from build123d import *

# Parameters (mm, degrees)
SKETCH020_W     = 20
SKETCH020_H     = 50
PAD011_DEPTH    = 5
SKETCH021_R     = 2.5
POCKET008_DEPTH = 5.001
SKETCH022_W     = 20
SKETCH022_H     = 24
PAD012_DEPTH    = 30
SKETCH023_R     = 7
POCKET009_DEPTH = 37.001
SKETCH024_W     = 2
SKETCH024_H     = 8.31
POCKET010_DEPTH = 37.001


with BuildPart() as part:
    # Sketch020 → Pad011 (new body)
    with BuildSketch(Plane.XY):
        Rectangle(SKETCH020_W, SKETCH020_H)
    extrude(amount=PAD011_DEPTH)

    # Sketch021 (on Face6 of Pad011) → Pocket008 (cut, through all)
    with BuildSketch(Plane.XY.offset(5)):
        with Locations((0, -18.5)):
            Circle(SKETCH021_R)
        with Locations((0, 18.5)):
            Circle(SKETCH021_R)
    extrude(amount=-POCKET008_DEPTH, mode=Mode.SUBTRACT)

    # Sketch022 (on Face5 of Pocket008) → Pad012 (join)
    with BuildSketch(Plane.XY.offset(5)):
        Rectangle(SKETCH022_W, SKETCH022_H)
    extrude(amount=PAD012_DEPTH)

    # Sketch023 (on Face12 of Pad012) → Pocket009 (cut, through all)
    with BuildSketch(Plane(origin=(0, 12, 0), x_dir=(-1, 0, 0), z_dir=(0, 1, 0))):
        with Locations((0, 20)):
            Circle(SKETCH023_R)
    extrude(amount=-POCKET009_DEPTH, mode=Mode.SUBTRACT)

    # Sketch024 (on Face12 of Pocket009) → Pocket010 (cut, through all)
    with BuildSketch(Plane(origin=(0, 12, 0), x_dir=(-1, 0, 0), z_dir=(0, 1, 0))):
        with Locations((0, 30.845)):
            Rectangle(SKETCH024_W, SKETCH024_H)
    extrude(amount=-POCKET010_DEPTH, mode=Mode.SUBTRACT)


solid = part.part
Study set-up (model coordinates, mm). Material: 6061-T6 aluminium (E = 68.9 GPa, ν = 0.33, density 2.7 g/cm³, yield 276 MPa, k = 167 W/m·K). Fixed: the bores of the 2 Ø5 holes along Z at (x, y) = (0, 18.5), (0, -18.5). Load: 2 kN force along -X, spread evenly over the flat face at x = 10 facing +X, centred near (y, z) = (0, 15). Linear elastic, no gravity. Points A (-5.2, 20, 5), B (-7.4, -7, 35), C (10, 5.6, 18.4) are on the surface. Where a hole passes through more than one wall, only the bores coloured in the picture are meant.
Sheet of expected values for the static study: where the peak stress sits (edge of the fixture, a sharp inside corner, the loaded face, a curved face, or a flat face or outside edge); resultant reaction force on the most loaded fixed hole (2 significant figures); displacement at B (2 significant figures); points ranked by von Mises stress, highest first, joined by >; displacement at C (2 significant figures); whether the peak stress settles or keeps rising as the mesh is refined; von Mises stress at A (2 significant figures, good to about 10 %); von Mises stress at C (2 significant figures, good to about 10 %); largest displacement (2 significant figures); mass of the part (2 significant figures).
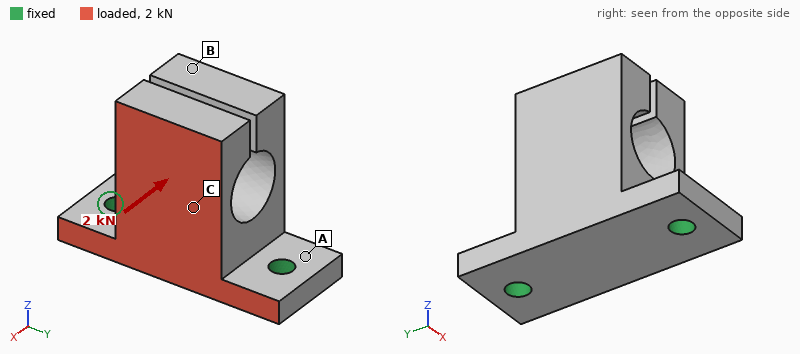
edge of the fixture
1.0 kN
0.14 mm
C > A > B
0.11 mm
keeps rising
51 MPa
140 MPa
0.36 mm
41 g
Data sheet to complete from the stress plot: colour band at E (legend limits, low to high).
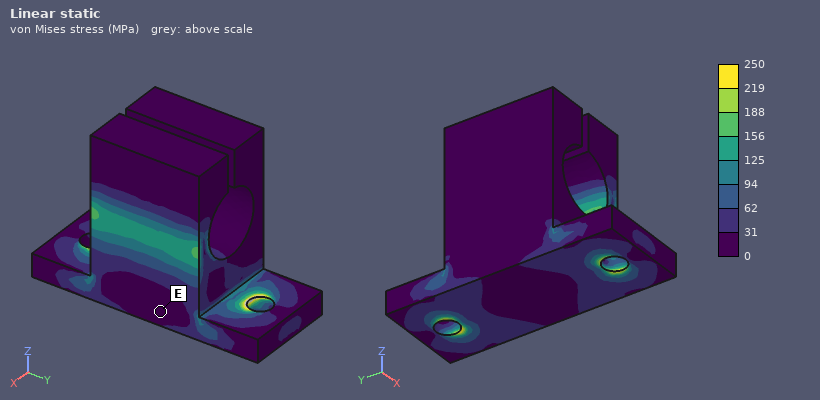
0 to 31 MPa
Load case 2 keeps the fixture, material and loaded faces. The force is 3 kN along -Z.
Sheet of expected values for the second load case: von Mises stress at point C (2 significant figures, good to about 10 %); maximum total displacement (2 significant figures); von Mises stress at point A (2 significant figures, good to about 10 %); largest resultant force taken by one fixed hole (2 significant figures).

57 MPa
0.23 mm
42 MPa
1.6 kN
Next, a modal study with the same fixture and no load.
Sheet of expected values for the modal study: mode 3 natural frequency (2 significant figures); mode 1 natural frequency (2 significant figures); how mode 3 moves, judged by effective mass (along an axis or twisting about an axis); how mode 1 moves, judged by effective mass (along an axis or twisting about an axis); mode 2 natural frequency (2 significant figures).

7800 Hz
2800 Hz
along Y
along X
3900 Hz
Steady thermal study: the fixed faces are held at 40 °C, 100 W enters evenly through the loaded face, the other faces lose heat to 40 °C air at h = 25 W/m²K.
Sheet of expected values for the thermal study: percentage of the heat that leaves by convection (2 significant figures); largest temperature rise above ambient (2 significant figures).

4.0 %
79 K
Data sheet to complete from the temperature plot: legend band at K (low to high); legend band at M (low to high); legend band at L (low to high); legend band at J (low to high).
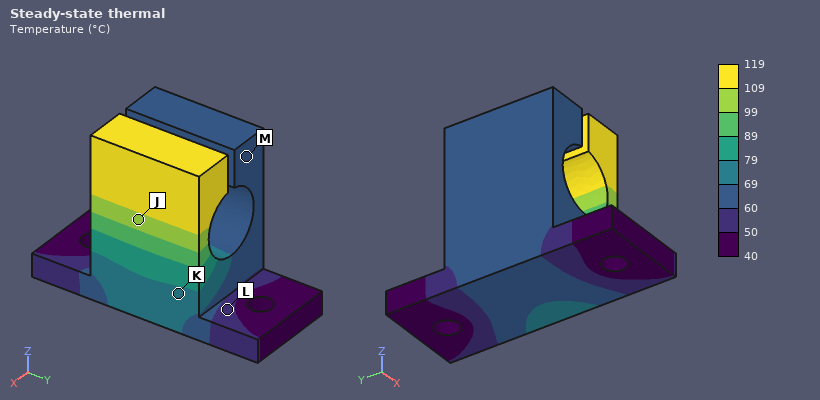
69 to 79 °C
60 to 69 °C
50 to 60 °C
99 to 109 °C
